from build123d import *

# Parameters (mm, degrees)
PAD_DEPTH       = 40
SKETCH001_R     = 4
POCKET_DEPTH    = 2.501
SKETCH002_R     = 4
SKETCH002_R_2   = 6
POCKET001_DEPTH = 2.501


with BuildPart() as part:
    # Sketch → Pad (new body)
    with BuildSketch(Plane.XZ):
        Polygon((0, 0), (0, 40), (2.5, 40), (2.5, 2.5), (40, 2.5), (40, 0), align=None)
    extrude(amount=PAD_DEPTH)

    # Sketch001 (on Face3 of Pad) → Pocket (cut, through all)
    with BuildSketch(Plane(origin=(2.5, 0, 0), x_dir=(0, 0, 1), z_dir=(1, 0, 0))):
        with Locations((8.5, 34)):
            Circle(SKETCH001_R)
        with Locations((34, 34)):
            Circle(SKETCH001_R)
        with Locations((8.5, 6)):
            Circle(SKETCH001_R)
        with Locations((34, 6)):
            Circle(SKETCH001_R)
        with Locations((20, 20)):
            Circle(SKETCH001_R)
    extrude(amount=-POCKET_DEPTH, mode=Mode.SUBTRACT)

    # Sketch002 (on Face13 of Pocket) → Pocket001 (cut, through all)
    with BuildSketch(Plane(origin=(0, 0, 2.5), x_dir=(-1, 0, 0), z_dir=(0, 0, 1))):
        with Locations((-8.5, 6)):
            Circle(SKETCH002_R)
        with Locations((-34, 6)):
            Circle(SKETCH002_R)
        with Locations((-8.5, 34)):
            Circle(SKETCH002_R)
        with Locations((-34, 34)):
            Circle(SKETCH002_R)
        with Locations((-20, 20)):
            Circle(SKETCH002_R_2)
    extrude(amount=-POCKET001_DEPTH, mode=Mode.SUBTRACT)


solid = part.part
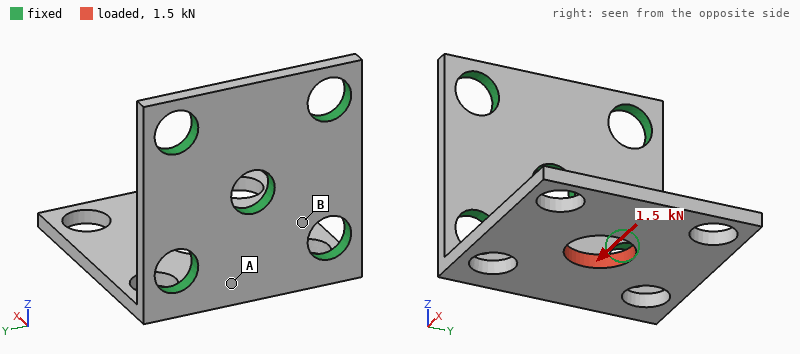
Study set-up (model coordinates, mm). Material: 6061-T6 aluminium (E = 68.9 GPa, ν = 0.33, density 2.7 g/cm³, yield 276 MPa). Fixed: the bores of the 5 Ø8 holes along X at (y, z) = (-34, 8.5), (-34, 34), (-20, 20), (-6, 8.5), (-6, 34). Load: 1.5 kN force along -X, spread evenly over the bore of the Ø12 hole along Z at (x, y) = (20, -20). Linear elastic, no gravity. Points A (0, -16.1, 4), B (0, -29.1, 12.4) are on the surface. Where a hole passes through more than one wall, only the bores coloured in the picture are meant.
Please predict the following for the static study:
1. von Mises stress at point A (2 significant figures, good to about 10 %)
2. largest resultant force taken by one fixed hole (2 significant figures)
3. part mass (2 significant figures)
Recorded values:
35 MPa
790 N
17 g
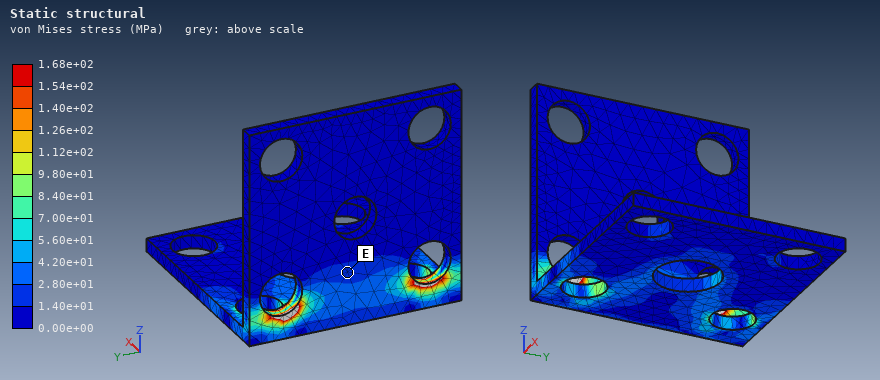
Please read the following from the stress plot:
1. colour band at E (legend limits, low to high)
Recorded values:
1.40e+01 to 2.80e+01 MPa
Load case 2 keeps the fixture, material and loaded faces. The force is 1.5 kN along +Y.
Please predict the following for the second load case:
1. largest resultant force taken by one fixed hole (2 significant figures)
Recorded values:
1.2 kN
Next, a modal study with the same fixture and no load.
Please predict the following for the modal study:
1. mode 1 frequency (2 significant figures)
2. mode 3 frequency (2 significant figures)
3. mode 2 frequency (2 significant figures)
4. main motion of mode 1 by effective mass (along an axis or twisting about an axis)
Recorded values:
1100 Hz
6900 Hz
2900 Hz
along Z
